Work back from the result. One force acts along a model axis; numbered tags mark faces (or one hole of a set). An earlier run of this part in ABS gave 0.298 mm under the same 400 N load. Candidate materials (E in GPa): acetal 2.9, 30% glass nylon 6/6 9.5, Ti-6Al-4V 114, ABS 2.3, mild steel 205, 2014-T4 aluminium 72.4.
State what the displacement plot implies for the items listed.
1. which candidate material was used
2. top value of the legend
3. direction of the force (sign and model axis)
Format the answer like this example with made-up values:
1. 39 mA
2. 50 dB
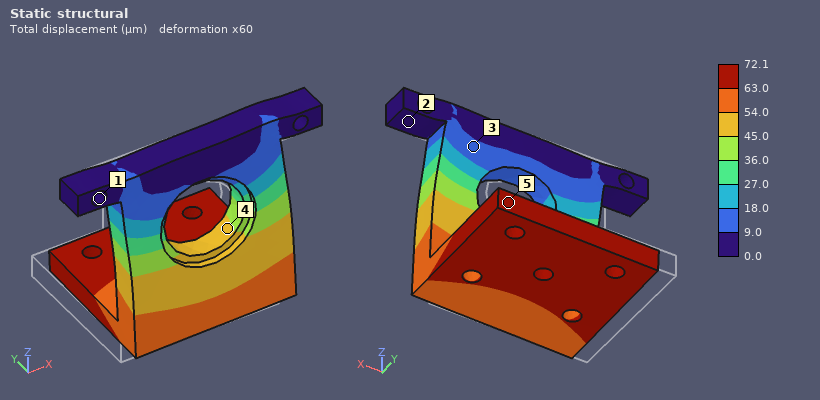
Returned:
1. 30% glass nylon 6/6
2. 72.1 µm
3. +X
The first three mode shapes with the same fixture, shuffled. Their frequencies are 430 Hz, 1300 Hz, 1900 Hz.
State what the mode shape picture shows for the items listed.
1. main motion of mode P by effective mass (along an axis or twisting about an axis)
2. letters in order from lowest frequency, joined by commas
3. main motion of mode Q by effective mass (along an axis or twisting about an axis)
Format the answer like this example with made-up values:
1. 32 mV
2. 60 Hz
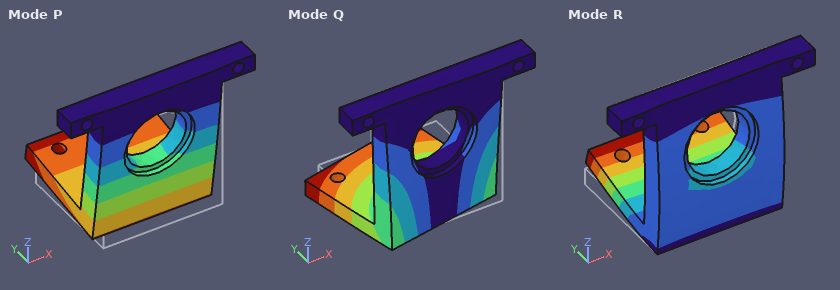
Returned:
1. along Y
2. P, Q, R
3. along X
